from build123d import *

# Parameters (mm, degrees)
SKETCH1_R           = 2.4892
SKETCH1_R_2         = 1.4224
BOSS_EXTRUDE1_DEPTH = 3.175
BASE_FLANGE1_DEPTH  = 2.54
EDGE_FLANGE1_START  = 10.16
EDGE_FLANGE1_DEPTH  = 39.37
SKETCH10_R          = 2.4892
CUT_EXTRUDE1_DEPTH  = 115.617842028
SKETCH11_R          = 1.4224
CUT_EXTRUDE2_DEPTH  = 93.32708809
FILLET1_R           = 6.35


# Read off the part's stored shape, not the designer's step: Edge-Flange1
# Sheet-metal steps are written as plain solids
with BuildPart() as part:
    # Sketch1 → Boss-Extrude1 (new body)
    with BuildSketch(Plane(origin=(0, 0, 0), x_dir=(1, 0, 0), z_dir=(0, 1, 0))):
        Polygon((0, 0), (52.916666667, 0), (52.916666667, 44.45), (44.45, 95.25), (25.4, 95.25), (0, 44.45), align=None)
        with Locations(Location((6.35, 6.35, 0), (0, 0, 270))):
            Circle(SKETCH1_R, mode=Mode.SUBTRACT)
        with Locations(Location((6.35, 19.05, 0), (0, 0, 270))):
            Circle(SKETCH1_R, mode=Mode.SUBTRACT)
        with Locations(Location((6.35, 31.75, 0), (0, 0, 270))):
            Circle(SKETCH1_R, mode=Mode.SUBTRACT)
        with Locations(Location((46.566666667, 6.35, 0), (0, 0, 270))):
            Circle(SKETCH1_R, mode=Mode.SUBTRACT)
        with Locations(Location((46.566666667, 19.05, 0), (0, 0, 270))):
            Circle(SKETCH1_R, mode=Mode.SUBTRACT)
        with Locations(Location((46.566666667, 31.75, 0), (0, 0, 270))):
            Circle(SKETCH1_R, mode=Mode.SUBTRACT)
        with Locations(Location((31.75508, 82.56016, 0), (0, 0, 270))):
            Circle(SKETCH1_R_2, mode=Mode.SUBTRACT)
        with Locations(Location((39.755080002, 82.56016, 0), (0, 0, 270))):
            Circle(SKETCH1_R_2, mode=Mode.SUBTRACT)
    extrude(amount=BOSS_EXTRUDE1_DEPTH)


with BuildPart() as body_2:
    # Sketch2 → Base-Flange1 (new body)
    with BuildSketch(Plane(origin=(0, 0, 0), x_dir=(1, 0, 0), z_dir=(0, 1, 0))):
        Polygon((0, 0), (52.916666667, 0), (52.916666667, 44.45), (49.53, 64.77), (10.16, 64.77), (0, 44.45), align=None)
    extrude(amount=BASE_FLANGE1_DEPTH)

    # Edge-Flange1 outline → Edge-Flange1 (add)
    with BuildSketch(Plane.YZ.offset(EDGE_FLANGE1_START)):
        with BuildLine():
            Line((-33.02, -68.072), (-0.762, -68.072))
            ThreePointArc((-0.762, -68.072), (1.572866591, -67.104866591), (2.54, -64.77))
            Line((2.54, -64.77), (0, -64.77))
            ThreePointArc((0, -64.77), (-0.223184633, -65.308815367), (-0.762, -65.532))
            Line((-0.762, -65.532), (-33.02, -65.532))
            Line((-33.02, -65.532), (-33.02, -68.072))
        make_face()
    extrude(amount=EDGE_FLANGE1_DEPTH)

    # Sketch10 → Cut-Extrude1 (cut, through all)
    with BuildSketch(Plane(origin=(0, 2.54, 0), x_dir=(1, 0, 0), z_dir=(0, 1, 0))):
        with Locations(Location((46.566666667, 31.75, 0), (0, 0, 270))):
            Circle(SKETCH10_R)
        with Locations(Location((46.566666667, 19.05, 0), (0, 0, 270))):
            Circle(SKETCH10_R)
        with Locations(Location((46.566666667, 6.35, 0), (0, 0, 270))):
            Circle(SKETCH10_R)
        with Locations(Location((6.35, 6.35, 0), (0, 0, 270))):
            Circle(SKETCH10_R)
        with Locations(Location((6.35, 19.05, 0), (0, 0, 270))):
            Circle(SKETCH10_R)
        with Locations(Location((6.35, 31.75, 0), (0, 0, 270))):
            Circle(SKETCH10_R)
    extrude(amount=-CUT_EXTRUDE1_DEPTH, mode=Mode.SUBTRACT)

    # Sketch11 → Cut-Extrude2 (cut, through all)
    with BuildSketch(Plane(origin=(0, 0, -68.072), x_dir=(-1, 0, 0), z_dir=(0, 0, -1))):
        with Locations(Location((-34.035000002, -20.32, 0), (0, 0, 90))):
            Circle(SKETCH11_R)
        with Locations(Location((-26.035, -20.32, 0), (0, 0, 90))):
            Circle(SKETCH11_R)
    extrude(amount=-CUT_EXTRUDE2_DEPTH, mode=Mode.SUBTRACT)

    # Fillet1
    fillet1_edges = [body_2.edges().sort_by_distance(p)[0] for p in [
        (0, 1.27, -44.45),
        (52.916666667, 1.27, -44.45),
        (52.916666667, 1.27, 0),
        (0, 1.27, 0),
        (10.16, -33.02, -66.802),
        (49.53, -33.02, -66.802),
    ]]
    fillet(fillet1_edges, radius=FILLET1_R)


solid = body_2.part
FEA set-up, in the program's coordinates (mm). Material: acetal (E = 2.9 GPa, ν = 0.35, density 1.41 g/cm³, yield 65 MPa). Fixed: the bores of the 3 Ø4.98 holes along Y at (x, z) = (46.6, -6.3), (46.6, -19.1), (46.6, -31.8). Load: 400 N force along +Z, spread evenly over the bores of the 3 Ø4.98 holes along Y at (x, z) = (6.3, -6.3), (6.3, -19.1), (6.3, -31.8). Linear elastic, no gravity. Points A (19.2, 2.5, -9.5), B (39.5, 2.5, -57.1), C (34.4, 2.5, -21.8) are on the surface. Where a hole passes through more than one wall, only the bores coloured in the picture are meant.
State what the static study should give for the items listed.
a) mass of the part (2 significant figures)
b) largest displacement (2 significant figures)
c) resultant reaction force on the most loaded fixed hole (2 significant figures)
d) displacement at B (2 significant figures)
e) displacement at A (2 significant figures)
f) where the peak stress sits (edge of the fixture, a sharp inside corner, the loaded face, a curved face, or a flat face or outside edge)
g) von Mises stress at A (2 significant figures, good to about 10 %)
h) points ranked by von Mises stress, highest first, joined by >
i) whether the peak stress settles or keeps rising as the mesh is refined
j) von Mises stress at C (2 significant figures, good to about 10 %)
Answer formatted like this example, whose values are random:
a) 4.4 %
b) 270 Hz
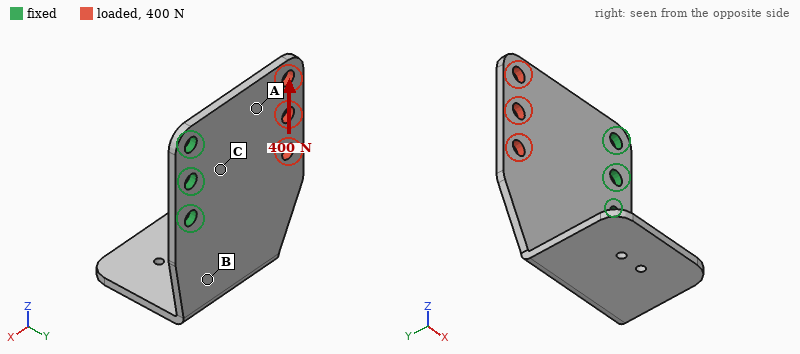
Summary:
a) 16 g
b) 0.51 mm
c) 570 N
d) 0.28 mm
e) 0.25 mm
f) edge of the fixture
g) 7.3 MPa
h) C > A > B
i) keeps rising
j) 12 MPa
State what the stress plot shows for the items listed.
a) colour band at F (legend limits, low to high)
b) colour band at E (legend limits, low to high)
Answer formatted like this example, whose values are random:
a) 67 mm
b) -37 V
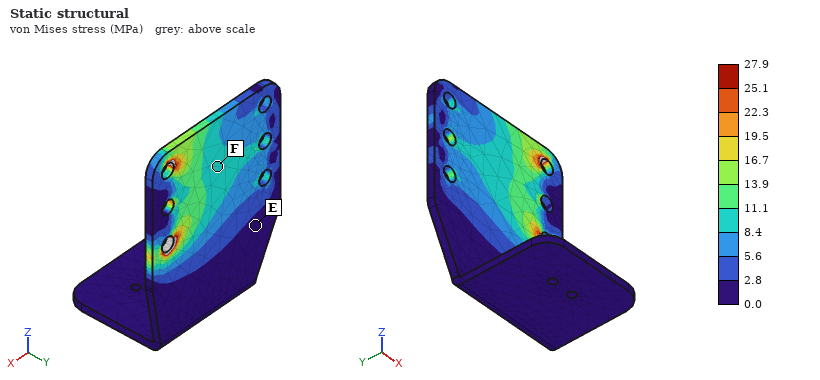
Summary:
a) 8.4 to 11.1 MPa
b) 0.0 to 2.8 MPa
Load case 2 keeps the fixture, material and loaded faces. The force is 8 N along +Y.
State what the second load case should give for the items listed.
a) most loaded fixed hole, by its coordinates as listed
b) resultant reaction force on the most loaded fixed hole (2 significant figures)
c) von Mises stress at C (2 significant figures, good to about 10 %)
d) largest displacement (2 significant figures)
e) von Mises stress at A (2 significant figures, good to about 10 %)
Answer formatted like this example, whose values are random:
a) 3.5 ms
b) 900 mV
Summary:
a) (46.6, -19.1)
b) 3.8 N
c) 3.6 MPa
d) 0.94 mm
e) 1.8 MPa
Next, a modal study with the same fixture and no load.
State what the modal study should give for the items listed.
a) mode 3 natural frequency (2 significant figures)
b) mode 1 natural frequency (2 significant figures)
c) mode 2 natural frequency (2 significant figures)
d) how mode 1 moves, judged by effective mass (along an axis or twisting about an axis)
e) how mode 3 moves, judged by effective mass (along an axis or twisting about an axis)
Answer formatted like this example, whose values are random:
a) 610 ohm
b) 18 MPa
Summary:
a) 440 Hz
b) 150 Hz
c) 230 Hz
d) along Y
e) along Y
